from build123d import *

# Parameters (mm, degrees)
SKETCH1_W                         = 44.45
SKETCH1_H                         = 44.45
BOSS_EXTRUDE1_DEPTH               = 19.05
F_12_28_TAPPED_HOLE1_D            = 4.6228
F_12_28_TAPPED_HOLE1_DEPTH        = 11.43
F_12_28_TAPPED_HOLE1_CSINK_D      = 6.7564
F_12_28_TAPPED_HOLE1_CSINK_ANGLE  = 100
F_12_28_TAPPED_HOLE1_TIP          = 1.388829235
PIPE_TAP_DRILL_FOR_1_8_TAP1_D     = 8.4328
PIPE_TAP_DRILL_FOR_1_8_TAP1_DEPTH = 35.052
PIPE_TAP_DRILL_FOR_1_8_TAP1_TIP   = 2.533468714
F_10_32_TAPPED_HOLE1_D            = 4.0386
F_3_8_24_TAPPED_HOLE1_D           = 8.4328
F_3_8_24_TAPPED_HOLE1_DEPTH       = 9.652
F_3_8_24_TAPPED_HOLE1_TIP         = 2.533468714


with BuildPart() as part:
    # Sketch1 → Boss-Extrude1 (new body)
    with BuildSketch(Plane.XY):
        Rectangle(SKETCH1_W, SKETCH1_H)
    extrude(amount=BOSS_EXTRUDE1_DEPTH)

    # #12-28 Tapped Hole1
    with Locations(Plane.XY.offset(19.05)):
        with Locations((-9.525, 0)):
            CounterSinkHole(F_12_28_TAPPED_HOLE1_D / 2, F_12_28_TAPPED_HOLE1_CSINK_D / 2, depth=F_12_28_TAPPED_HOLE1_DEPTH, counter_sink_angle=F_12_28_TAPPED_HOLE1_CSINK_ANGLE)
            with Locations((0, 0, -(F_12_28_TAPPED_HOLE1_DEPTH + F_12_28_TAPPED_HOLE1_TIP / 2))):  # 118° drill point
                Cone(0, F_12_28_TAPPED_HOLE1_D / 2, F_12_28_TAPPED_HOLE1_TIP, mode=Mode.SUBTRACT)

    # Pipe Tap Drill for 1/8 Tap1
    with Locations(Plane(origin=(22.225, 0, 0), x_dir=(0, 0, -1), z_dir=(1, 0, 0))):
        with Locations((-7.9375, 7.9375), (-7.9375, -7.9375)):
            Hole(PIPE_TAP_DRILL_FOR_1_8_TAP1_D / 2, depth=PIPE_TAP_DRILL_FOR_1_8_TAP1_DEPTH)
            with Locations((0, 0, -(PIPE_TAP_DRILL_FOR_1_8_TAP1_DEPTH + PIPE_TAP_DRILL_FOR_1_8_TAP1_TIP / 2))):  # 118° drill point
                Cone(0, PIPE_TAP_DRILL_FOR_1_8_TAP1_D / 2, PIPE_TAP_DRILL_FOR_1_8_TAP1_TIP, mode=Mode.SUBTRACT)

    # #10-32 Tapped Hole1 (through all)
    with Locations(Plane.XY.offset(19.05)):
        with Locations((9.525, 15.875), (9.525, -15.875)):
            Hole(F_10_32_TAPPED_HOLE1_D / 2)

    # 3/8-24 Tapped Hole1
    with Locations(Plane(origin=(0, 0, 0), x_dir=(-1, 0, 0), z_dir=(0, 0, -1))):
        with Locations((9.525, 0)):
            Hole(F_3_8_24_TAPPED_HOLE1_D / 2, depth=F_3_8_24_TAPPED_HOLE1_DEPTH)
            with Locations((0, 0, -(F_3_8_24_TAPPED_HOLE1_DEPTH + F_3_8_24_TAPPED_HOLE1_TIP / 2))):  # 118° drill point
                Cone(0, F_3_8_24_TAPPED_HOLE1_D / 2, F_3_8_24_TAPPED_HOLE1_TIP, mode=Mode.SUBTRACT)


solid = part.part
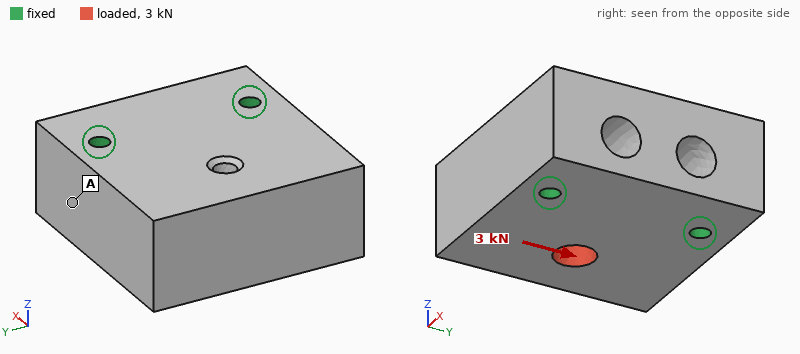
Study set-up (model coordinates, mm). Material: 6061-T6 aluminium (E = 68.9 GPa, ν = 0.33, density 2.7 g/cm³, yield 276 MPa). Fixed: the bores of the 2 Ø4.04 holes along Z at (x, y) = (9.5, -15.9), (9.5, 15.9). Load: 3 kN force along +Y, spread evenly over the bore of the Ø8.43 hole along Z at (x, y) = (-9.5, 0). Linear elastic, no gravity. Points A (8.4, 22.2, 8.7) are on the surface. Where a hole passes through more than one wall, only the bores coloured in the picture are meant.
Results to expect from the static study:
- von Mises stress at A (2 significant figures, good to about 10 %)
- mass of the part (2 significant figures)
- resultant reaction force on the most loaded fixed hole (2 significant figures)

10 MPa
88 g
2.2 kN
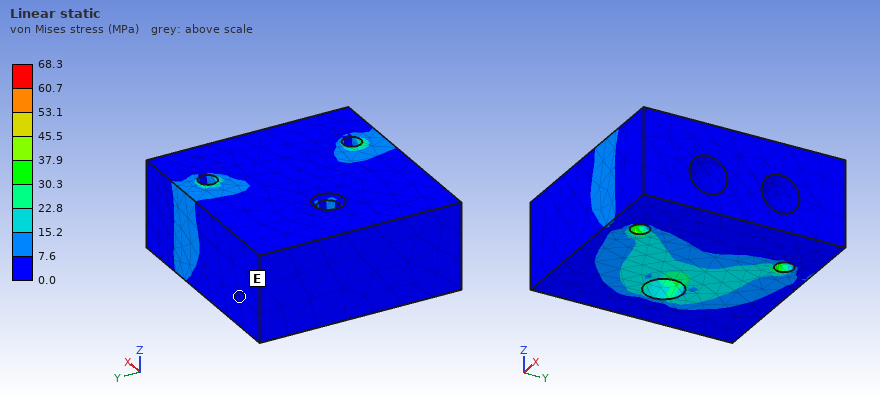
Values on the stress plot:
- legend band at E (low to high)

0.0 to 7.6 MPa
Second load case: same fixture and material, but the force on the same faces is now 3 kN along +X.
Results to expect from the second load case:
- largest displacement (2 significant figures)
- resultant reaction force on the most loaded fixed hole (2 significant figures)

8.9 µm
1.5 kN
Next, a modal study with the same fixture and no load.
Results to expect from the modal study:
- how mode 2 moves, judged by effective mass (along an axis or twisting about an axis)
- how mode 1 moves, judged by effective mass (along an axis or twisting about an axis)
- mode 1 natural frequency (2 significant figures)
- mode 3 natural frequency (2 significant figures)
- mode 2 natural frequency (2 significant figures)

along Y
along Z
10 kHz
18 kHz
16 kHz
